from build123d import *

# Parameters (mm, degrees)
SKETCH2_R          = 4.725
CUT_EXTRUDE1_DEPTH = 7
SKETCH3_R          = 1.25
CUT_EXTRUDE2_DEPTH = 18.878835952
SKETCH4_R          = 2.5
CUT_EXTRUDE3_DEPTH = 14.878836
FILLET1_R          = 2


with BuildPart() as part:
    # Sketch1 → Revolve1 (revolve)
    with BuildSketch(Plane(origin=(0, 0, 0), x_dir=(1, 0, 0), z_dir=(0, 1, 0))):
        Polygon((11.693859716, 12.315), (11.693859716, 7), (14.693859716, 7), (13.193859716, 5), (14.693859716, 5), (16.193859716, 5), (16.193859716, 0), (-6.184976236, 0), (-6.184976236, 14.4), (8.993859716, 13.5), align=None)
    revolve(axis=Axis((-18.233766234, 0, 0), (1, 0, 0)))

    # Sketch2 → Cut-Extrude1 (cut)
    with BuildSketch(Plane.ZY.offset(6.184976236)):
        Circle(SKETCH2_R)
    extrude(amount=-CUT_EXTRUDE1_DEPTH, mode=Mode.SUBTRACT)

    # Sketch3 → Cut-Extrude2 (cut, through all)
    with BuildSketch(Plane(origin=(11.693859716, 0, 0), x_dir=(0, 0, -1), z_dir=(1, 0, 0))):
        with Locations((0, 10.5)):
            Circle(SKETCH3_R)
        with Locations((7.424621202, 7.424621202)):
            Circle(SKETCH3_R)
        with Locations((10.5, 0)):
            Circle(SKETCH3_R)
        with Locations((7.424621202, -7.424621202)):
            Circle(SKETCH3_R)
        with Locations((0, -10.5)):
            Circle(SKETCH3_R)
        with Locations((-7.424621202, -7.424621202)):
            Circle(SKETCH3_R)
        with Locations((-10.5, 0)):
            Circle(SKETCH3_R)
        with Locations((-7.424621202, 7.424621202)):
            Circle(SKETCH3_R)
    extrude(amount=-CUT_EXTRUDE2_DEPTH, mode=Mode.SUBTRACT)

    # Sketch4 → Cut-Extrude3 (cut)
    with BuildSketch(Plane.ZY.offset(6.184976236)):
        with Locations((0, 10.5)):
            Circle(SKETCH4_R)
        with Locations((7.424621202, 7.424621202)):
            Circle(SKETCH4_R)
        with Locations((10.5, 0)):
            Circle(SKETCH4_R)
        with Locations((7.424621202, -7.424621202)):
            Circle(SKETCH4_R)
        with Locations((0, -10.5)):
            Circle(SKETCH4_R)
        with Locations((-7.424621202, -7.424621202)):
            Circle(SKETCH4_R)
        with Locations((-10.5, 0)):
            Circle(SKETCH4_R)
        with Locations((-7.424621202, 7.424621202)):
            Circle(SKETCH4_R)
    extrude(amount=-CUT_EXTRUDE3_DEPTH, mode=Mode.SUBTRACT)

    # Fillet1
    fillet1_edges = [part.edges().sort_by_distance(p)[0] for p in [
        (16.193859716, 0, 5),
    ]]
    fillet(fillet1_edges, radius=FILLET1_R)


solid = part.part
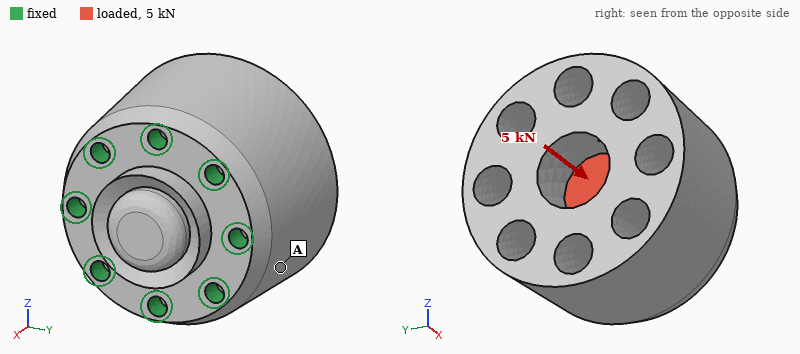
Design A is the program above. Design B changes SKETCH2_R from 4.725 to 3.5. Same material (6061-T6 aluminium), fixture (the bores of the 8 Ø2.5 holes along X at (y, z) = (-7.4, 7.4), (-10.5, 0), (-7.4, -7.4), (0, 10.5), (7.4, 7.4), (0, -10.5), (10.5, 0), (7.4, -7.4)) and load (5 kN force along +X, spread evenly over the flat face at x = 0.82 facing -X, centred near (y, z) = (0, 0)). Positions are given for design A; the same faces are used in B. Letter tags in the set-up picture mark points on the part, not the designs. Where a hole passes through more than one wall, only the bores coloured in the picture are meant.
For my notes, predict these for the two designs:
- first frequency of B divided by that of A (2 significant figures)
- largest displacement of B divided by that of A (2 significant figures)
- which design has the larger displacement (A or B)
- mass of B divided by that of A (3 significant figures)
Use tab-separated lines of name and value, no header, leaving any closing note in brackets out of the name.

first frequency of B divided by that of A	0.98
largest displacement of B divided by that of A	1.3
which design has the larger displacement	B
mass of B divided by that of A	1.03
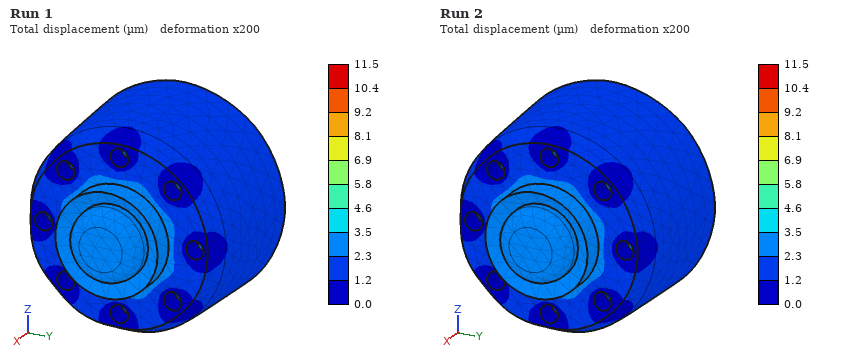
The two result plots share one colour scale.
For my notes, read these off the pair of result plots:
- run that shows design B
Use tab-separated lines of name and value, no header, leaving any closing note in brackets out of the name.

run that shows design B	Run 1
